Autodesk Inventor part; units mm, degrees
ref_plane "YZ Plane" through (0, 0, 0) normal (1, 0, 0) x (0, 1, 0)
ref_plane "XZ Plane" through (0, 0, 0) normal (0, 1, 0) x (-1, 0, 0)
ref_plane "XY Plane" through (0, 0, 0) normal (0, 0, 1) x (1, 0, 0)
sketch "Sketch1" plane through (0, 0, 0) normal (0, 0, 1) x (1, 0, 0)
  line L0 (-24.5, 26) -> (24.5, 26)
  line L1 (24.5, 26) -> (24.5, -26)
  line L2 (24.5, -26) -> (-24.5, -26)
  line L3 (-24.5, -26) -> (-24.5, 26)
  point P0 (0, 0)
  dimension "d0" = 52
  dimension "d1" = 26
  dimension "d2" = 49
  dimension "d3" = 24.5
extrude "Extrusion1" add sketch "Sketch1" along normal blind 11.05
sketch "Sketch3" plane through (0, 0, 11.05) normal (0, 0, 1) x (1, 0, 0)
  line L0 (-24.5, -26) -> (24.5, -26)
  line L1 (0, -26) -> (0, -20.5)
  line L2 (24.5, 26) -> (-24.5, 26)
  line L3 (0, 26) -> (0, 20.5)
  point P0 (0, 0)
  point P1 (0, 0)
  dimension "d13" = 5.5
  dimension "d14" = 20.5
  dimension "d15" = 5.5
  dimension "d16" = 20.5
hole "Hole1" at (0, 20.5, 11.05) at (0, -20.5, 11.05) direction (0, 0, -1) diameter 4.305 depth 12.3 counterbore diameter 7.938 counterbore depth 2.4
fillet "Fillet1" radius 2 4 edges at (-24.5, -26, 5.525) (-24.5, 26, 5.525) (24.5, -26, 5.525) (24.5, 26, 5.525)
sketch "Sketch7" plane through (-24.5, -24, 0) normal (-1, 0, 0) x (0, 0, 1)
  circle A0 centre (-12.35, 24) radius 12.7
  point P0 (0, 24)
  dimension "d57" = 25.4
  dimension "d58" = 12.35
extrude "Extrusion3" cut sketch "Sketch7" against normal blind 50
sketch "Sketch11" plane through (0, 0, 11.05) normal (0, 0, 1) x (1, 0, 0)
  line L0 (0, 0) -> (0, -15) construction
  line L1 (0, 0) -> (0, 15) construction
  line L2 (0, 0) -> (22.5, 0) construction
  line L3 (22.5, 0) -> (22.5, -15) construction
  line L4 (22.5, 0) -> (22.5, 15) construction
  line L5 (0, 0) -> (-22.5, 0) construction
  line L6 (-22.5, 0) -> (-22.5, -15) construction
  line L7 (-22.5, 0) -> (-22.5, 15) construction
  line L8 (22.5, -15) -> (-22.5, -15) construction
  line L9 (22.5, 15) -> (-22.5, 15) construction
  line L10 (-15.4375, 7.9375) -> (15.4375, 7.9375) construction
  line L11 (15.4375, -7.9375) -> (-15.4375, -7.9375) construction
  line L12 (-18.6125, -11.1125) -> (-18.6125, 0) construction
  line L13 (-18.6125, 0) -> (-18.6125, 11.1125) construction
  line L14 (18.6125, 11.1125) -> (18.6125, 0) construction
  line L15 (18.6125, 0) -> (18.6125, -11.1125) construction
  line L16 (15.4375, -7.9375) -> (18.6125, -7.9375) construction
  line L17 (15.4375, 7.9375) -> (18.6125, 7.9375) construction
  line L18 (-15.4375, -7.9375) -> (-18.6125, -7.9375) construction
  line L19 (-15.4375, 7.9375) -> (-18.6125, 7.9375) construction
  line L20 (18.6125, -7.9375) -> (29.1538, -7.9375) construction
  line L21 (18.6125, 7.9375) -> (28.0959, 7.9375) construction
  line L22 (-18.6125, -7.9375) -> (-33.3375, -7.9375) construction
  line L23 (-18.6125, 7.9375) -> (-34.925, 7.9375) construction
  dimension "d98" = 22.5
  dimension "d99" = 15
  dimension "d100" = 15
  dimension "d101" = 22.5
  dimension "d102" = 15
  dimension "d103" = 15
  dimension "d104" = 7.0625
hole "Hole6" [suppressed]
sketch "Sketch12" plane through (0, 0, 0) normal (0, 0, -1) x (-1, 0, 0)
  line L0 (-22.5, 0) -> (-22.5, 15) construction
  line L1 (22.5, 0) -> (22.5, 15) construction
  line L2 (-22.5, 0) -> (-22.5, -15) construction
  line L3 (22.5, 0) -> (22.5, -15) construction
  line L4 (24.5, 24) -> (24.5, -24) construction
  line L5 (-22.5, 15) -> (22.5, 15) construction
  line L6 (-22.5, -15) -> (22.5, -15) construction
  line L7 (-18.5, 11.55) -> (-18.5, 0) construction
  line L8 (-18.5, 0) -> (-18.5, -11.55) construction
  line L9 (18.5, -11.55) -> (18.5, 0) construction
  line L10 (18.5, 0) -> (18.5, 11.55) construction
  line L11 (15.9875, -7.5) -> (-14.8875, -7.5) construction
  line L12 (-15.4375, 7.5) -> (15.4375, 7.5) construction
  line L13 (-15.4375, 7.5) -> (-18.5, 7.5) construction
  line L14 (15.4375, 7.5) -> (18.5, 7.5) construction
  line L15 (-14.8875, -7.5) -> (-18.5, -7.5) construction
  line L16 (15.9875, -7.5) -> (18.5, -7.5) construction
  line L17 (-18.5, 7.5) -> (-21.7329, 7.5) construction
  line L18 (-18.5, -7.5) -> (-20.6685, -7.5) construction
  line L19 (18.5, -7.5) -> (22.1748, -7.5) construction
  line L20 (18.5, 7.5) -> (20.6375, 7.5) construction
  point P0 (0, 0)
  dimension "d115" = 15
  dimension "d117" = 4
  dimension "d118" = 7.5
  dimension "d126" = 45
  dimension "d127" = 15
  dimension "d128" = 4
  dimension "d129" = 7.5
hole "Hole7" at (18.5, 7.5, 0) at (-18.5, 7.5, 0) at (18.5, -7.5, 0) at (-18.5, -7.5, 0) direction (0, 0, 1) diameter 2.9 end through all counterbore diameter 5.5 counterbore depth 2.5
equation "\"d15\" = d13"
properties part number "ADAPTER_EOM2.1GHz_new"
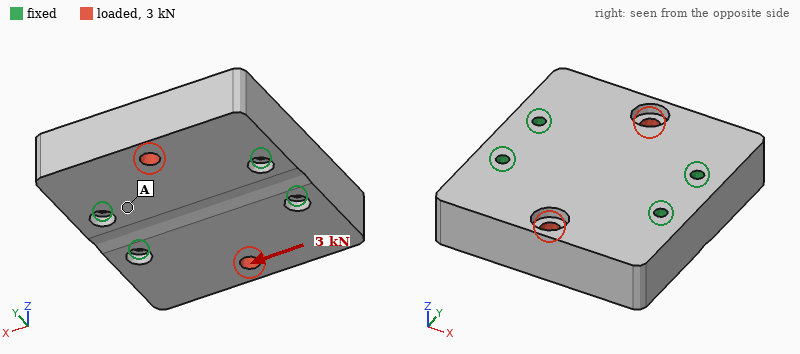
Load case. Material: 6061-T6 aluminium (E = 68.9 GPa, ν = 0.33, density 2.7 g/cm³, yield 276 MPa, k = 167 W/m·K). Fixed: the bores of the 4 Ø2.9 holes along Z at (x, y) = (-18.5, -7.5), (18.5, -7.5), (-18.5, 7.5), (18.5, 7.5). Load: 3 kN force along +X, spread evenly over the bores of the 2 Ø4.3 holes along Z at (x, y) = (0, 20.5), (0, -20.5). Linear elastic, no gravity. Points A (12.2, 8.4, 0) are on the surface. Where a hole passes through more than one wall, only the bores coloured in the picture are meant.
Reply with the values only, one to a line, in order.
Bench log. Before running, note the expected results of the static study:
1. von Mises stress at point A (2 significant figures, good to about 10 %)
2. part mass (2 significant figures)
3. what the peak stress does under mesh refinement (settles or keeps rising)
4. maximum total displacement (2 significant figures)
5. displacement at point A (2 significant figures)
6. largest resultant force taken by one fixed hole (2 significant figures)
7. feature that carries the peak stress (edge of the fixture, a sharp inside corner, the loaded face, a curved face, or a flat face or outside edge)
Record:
3.8 MPa
73 g
keeps rising
3.6 µm
0.73 µm
800 N
edge of the fixture
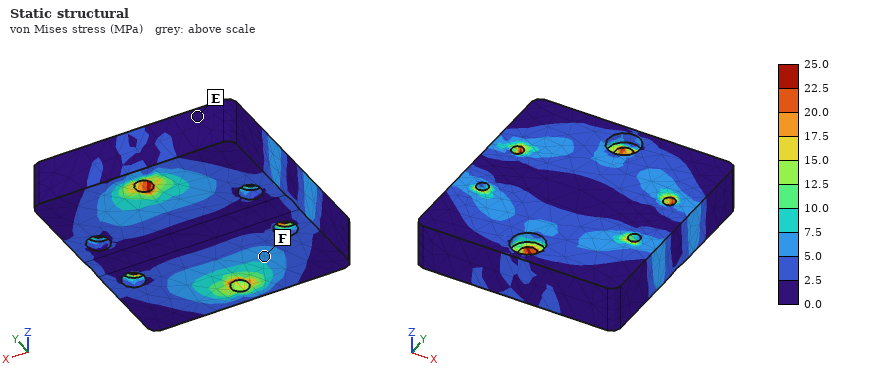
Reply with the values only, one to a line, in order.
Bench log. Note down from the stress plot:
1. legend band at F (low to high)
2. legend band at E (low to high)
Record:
5.0 to 7.5 MPa
0.0 to 2.5 MPa
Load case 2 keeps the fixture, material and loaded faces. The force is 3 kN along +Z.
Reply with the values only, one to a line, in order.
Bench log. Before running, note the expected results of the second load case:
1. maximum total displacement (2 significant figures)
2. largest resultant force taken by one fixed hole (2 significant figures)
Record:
22 µm
820 N
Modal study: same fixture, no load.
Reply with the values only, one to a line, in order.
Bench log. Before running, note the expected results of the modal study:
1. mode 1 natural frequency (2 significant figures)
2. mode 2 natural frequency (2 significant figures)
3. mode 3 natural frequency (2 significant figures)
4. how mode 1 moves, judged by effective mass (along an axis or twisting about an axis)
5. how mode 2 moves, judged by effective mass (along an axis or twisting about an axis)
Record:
13 kHz
14 kHz
21 kHz
twisting about X
along Z
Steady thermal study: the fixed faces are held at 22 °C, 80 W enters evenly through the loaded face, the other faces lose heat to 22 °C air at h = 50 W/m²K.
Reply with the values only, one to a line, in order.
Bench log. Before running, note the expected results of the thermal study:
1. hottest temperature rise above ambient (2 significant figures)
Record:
19 K
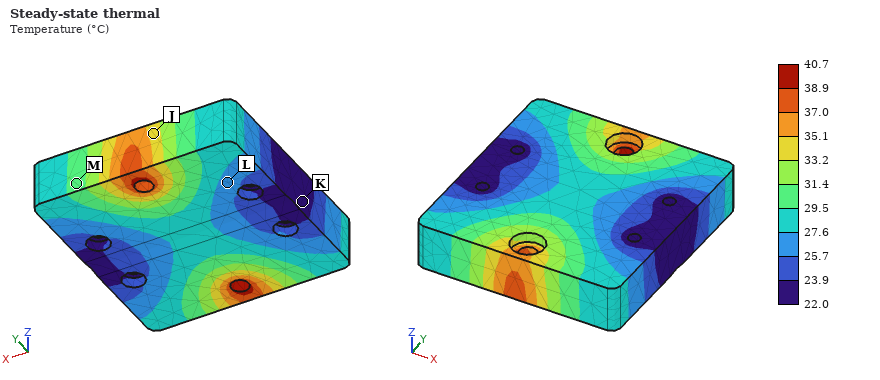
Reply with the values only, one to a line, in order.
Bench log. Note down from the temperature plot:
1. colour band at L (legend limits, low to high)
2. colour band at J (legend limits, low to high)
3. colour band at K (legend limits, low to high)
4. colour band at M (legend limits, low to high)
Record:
25.7 to 27.6 °C
33.2 to 35.1 °C
22.0 to 23.9 °C
29.5 to 31.4 °C
